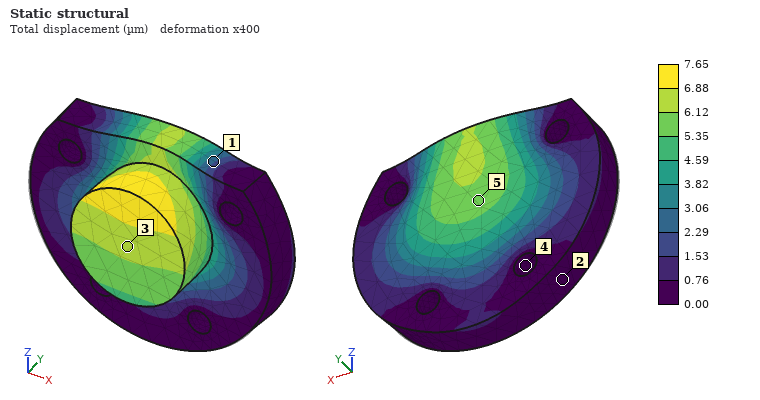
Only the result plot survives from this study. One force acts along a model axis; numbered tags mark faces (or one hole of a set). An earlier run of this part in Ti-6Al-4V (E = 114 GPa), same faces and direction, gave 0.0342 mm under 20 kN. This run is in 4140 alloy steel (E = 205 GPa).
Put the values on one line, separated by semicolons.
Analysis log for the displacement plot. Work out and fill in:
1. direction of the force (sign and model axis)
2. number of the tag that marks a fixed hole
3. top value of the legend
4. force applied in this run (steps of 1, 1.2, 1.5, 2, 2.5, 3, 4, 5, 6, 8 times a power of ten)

+Y; 4; 7.65 µm; 8 kN
